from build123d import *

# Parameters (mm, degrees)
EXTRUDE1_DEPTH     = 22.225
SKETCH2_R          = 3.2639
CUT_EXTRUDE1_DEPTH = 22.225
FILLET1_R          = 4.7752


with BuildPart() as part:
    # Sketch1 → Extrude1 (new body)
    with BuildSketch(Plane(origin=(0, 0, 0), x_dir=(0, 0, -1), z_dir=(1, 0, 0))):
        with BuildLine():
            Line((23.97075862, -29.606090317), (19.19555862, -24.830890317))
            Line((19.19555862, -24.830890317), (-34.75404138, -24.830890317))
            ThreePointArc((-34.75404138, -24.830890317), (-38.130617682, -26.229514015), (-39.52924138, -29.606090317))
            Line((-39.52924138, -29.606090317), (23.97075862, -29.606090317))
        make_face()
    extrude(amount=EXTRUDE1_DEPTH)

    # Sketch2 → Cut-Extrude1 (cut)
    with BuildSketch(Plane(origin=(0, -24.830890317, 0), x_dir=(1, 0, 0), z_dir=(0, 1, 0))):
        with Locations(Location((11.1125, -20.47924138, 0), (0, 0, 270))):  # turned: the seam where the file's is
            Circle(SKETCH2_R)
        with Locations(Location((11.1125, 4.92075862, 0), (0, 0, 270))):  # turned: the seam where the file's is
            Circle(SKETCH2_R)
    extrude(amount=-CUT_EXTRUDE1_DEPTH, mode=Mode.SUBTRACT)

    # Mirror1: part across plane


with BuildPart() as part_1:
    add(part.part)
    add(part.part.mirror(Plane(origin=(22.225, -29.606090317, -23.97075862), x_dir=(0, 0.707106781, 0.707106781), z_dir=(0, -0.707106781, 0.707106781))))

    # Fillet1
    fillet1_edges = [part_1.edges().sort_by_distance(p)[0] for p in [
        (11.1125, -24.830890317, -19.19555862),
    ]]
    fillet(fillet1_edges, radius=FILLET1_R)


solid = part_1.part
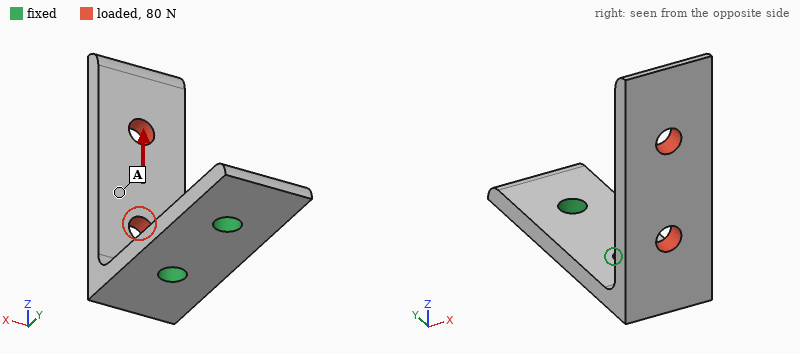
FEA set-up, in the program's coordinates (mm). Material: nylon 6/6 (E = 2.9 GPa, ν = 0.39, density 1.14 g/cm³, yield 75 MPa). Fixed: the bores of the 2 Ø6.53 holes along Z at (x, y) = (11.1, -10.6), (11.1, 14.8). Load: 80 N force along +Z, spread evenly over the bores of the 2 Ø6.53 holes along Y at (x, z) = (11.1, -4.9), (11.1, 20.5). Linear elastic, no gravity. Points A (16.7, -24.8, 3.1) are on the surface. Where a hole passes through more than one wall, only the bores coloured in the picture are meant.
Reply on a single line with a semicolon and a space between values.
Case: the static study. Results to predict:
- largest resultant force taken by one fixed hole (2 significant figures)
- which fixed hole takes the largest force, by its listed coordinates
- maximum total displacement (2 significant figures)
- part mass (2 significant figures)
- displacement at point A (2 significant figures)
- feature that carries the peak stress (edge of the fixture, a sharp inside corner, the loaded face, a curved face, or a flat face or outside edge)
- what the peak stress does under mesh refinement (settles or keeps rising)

85 N; (11.1, -10.6); 0.92 mm; 14 g; 0.38 mm; edge of the fixture; keeps rising
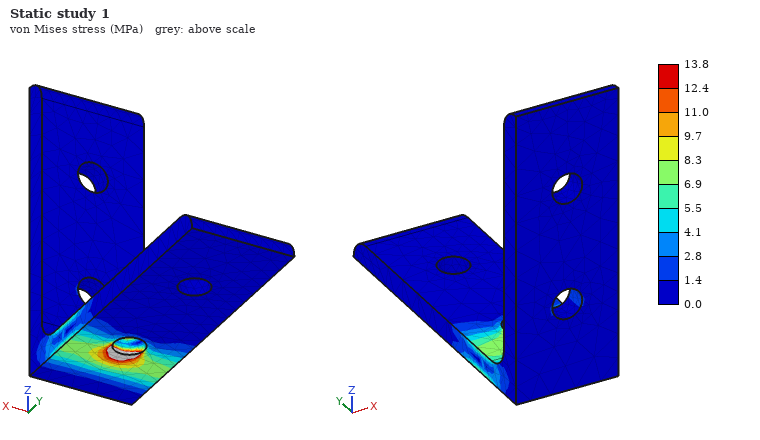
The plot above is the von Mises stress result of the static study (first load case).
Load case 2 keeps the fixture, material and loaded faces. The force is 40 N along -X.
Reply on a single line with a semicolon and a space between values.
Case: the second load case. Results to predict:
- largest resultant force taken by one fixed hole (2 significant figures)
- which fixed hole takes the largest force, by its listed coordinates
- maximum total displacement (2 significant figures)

53 N; (11.1, -10.6); 0.97 mm
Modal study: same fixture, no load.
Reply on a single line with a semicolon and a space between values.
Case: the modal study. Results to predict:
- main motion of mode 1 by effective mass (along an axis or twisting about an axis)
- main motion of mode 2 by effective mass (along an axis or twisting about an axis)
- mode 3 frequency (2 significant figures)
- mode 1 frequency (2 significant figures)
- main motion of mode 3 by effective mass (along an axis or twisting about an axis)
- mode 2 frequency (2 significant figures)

along Y; along X; 1300 Hz; 270 Hz; along Z; 460 Hz
